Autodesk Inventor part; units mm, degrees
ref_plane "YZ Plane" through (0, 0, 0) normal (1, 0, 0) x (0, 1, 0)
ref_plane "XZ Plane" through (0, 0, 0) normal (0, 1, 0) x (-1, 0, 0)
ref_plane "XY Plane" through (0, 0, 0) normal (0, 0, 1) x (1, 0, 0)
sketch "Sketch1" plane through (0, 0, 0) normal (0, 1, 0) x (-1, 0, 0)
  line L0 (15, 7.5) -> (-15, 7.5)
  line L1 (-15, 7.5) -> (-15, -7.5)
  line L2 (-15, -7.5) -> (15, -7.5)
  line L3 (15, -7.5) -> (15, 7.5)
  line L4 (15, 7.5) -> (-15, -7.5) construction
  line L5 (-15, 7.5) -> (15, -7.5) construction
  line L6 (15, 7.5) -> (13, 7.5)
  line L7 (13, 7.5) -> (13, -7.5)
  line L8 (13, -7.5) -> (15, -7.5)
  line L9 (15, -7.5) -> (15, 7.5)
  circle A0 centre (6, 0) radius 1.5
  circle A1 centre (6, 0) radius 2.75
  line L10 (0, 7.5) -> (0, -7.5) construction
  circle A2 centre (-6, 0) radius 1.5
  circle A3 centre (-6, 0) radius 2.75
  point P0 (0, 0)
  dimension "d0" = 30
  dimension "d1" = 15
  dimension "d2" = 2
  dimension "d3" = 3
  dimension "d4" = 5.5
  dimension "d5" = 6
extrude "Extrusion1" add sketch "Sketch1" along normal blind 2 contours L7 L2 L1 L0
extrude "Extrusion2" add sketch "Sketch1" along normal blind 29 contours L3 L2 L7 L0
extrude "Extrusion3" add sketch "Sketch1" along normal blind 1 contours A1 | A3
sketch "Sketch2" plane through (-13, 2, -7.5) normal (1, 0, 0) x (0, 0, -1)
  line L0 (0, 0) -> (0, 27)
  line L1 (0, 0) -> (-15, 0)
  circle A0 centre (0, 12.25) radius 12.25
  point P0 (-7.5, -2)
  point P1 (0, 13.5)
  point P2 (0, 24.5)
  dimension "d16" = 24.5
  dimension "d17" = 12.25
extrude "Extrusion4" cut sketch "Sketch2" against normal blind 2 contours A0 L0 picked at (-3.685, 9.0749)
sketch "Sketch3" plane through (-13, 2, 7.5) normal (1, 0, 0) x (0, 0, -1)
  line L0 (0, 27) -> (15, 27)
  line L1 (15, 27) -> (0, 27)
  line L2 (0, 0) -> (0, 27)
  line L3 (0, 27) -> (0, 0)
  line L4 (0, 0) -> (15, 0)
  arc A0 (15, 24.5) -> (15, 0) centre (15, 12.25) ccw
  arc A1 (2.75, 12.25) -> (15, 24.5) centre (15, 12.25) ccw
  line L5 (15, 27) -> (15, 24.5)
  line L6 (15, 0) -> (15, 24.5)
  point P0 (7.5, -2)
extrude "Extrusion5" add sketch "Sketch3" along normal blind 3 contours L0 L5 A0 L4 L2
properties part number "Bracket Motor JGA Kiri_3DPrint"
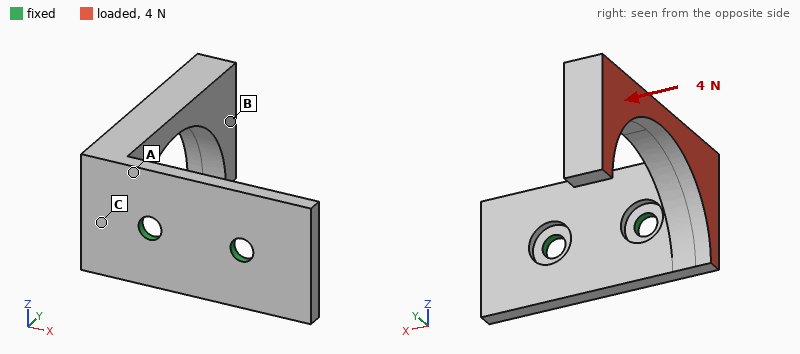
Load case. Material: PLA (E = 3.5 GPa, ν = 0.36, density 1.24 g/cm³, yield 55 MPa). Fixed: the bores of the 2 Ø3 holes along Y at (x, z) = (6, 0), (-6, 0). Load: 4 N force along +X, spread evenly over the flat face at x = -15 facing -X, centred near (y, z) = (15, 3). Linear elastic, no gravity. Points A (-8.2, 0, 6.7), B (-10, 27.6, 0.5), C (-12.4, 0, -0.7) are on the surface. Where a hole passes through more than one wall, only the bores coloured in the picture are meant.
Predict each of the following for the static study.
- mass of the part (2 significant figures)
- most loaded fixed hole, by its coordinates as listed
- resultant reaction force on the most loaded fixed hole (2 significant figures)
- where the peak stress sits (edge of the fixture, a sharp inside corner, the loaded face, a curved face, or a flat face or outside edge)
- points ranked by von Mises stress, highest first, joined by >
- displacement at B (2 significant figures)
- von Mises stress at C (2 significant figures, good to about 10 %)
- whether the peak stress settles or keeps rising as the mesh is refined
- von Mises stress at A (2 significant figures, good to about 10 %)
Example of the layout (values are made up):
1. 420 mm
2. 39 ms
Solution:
1. 2.1 g
2. (6, 0)
3. 9.8 N
4. edge of the fixture
5. A > C > B
6. 0.41 mm
7. 2.0 MPa
8. keeps rising
9. 5.6 MPa
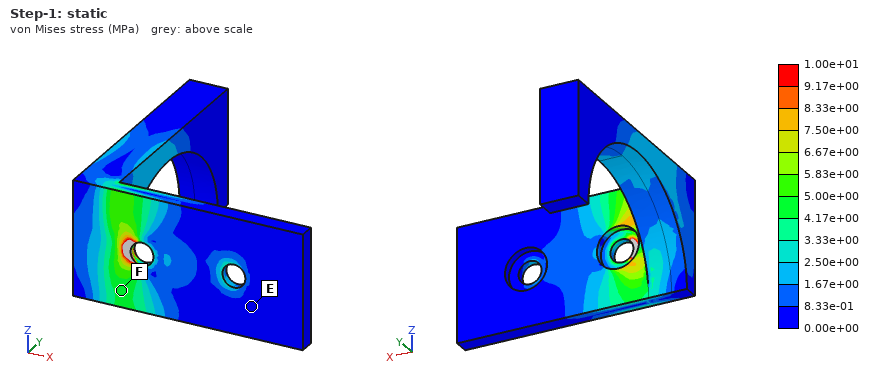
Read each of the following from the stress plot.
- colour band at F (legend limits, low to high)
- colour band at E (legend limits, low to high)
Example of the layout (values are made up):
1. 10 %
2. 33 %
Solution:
1. 4.17e+00 to 5.00e+00 MPa
2. 0.00e+00 to 8.33e-01 MPa
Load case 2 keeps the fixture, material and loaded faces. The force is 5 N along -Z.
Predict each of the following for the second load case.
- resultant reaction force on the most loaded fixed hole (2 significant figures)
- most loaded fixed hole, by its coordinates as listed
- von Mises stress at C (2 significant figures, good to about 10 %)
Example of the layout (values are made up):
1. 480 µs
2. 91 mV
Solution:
1. 6.7 N
2. (-6, 0)
3. 2.5 MPa
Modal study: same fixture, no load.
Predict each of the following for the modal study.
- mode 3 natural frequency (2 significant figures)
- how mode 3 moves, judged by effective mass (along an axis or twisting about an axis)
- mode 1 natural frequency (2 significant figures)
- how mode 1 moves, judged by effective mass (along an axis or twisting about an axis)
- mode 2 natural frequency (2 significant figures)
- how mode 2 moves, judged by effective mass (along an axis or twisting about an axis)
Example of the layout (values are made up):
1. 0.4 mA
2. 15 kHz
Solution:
1. 2000 Hz
2. along Y
3. 480 Hz
4. along X
5. 550 Hz
6. along Z
